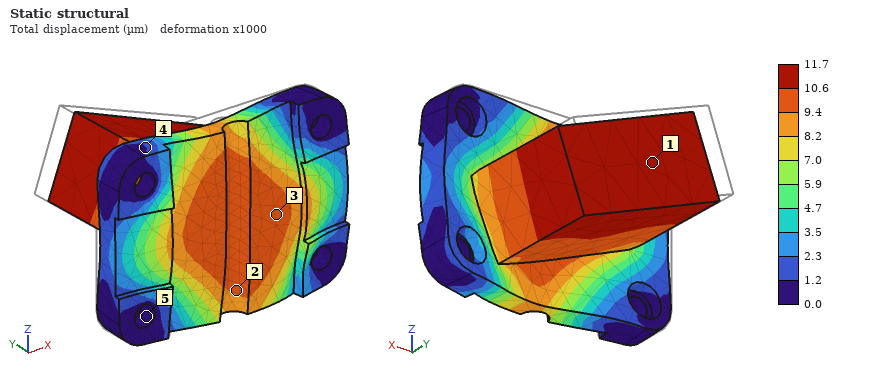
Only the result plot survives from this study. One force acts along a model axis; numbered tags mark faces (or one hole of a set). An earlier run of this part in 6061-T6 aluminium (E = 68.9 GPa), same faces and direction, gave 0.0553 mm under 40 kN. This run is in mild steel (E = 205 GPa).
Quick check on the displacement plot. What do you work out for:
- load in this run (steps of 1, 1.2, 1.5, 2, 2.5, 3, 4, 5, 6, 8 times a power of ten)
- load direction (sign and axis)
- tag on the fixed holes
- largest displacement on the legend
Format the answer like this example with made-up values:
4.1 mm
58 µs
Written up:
25 kN
-Y
5
11.7 µm
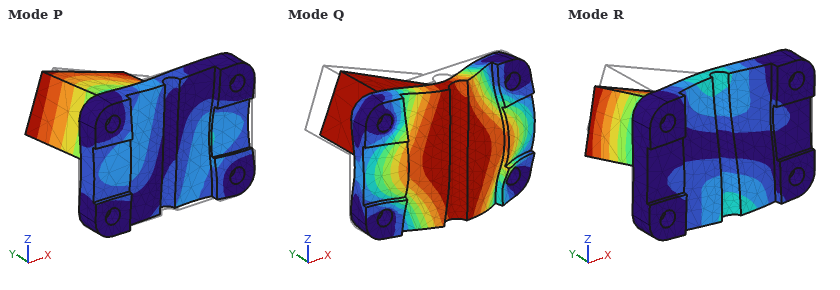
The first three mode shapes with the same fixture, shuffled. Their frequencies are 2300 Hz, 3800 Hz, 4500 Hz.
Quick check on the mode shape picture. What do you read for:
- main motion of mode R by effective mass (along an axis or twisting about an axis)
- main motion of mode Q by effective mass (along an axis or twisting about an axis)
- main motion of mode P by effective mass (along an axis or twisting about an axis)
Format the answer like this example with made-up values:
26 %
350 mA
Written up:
along Z
along Y
along X
